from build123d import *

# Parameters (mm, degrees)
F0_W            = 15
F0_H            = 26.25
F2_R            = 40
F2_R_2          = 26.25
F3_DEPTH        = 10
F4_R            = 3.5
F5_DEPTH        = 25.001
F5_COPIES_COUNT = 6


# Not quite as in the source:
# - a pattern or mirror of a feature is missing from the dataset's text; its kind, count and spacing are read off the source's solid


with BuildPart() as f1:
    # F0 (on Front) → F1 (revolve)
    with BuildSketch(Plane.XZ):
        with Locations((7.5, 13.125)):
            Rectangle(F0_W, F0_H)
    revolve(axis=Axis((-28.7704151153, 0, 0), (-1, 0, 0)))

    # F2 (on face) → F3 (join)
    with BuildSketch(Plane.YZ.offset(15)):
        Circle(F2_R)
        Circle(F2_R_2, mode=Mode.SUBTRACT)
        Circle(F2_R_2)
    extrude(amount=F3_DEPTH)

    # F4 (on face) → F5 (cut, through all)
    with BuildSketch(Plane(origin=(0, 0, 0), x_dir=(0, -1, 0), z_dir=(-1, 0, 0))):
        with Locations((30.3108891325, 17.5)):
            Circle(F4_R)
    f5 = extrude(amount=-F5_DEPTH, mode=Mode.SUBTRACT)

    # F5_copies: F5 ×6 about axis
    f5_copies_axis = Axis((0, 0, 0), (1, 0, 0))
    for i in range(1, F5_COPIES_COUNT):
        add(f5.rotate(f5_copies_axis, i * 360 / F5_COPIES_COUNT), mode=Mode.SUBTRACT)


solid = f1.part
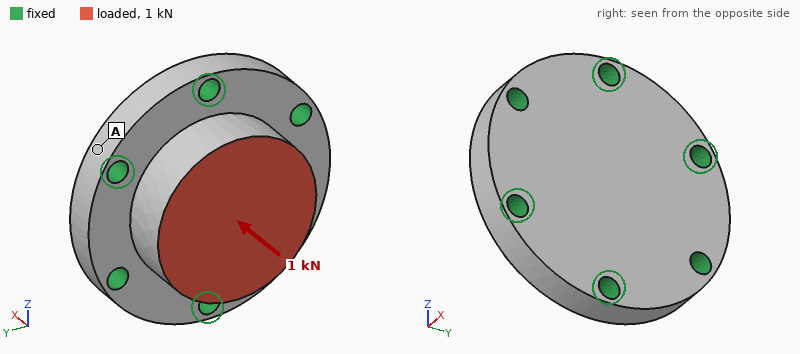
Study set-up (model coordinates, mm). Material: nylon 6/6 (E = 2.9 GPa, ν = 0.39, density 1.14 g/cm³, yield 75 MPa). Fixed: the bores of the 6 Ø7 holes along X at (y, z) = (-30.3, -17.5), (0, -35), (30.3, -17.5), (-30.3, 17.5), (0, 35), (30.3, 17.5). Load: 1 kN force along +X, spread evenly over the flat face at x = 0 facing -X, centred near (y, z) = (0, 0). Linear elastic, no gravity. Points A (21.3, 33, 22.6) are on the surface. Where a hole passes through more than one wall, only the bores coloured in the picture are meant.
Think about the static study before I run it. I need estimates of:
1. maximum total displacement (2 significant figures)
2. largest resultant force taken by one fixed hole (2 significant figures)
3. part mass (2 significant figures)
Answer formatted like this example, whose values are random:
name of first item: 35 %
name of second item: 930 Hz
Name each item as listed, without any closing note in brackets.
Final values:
maximum total displacement: 18 µm
largest resultant force taken by one fixed hole: 180 N
part mass: 92 g
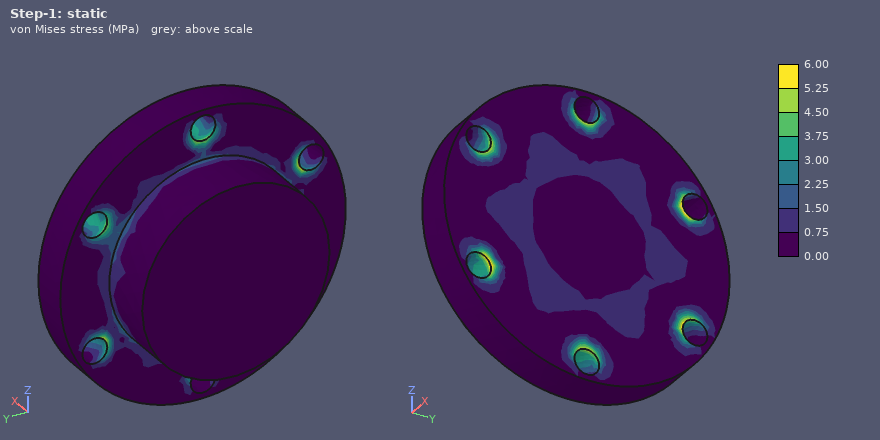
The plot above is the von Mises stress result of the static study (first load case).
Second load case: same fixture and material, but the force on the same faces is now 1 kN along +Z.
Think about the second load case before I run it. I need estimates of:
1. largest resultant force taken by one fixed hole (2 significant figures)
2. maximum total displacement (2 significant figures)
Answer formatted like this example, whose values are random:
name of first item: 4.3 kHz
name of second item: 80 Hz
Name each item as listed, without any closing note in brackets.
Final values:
largest resultant force taken by one fixed hole: 320 N
maximum total displacement: 30 µm
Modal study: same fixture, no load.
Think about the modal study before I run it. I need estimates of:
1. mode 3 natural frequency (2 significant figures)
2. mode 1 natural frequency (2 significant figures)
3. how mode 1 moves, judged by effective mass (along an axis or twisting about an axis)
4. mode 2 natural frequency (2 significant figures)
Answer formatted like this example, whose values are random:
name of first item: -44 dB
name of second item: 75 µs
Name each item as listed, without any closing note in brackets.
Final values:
mode 3 natural frequency: 6200 Hz
mode 1 natural frequency: 5000 Hz
how mode 1 moves, judged by effective mass: along X
mode 2 natural frequency: 6200 Hz
